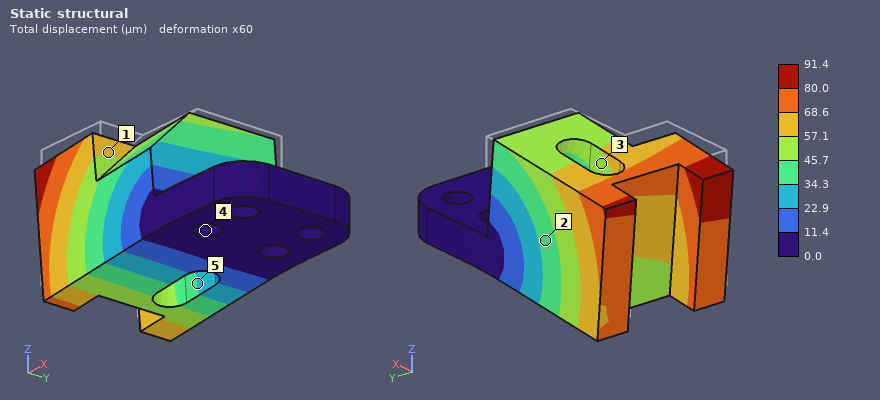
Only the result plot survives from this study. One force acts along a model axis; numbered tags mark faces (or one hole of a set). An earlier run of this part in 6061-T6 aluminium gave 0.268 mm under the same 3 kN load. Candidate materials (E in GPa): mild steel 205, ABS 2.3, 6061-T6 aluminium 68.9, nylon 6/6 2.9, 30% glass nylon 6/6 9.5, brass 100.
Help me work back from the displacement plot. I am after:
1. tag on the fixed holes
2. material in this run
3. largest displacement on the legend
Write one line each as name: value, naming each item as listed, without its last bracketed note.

tag on the fixed holes: 4
material in this run: mild steel
largest displacement on the legend: 91.4 µm
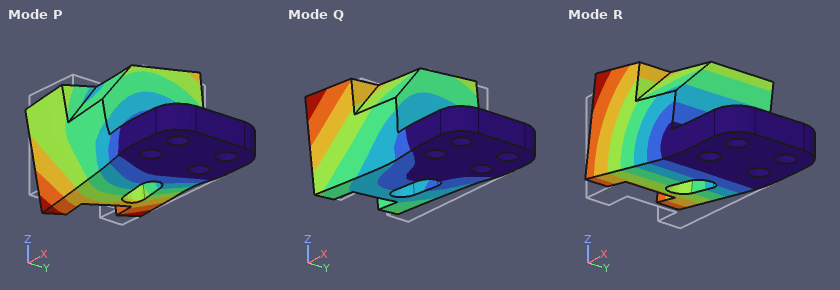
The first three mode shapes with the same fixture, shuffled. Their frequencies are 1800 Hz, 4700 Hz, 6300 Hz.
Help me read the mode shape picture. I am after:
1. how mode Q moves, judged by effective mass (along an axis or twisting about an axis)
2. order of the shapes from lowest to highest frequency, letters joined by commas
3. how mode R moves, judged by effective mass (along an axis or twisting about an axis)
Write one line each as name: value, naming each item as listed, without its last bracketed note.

how mode Q moves, judged by effective mass: along Y
order of the shapes from lowest to highest frequency, letters joined by commas: R, Q, P
how mode R moves, judged by effective mass: along Z
